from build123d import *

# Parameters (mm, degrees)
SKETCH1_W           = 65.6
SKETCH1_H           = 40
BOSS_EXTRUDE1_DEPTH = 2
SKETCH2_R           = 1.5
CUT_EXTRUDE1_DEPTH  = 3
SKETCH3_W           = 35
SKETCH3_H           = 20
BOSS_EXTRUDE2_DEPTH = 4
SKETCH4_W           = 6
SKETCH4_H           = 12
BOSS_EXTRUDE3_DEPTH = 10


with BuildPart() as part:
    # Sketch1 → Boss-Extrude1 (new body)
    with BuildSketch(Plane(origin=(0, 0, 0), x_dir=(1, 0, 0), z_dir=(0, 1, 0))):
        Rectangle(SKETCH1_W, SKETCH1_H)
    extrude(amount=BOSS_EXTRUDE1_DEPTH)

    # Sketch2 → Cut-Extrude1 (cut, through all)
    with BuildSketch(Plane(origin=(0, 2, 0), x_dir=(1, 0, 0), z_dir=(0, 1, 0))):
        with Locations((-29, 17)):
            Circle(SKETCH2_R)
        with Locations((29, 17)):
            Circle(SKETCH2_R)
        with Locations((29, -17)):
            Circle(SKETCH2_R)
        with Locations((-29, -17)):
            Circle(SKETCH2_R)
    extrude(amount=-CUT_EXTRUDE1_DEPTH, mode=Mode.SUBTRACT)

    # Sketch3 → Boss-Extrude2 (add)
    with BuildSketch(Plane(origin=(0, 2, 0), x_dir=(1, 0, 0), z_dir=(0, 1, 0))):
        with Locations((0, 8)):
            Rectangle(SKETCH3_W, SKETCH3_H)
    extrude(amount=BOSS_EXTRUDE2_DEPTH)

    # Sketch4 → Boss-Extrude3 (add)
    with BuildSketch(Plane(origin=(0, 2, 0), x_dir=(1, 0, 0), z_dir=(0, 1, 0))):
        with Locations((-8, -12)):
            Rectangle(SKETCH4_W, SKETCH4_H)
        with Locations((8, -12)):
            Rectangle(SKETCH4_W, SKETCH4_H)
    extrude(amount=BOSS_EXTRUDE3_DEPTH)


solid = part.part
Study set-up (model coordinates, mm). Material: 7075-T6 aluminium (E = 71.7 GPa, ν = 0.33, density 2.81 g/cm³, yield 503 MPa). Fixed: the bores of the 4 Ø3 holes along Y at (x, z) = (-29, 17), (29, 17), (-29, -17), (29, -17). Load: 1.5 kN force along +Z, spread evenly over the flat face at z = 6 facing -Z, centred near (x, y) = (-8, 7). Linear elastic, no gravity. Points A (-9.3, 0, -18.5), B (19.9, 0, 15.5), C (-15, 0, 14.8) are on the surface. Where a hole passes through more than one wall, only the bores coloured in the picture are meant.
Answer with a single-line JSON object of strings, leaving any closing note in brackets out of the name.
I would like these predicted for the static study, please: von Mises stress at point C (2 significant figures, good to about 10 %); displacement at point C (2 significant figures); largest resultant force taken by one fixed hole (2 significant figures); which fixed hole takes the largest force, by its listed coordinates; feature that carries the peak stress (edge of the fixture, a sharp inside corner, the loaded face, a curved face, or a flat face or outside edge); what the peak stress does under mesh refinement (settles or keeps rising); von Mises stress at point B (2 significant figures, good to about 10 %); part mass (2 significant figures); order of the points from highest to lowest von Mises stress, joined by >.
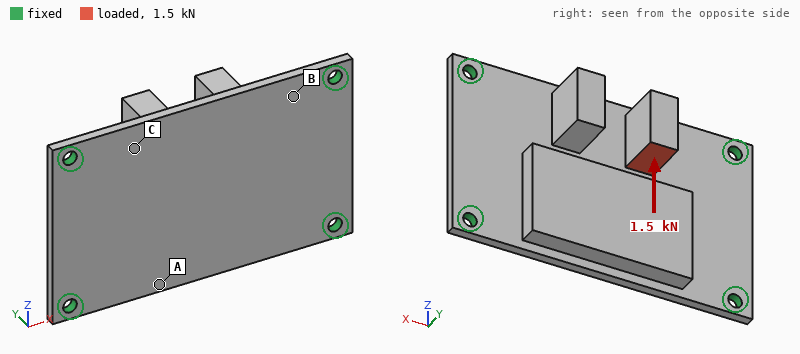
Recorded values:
{"von Mises stress at point C": "130 MPa", "displacement at point C": "0.15 mm", "largest resultant force taken by one fixed hole": "670 N", "which fixed hole takes the largest force, by its listed coordinates": "(-29, -17)", "feature that carries the peak stress": "edge of the fixture", "what the peak stress does under mesh refinement": "keeps rising", "von Mises stress at point B": "79 MPa", "part mass": "27 g", "order of the points from highest to lowest von Mises stress, joined by >": "C > B > A"}
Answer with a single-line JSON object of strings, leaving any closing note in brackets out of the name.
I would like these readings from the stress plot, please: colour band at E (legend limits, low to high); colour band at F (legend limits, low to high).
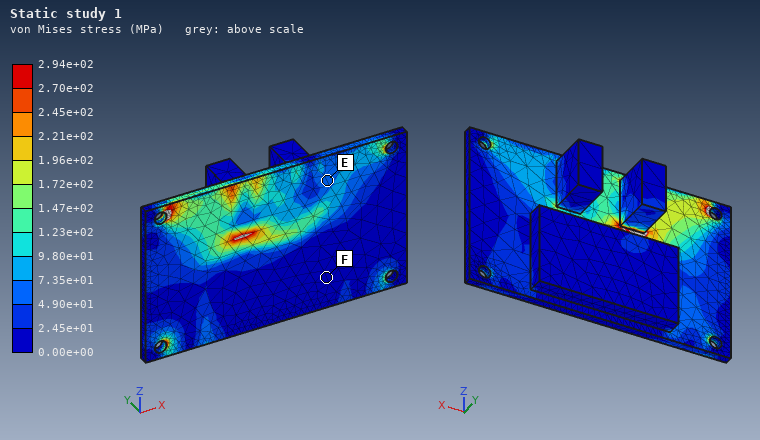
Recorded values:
{"colour band at E": "4.90e+01 to 7.35e+01 MPa", "colour band at F": "0.00e+00 to 2.45e+01 MPa"}
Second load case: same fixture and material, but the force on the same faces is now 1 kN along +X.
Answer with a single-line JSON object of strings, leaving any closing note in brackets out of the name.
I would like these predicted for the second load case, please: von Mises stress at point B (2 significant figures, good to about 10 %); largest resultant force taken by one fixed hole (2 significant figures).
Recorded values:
{"von Mises stress at point B": "29 MPa", "largest resultant force taken by one fixed hole": "330 N"}
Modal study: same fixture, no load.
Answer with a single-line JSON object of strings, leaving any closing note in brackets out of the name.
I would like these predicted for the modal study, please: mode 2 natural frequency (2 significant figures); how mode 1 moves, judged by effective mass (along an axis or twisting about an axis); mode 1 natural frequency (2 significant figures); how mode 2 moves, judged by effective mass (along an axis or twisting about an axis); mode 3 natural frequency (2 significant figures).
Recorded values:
{"mode 2 natural frequency": "4200 Hz", "how mode 1 moves, judged by effective mass": "along Y", "mode 1 natural frequency": "2700 Hz", "how mode 2 moves, judged by effective mass": "along Y", "mode 3 natural frequency": "6600 Hz"}
